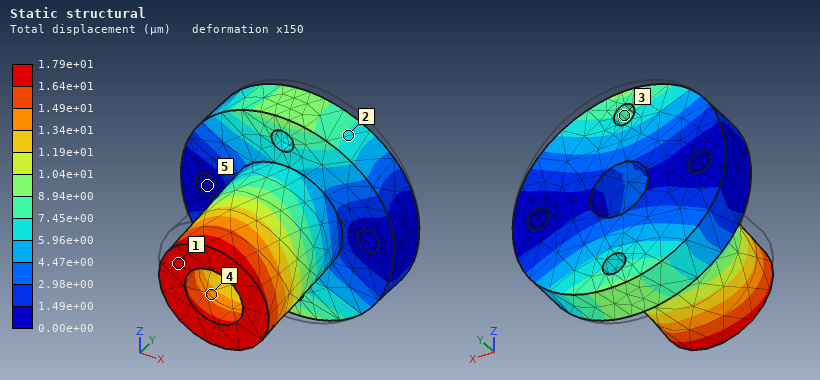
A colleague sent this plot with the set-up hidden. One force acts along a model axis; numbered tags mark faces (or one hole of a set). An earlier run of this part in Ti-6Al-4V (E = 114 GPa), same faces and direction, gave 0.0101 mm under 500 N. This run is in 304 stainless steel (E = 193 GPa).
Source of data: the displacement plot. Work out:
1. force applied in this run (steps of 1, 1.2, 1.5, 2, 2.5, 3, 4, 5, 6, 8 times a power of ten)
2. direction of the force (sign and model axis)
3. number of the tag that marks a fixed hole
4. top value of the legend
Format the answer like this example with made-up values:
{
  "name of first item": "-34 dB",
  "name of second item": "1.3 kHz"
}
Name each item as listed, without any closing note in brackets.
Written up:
{
  "force applied in this run": "1.5 kN",
  "direction of the force": "-Z",
  "number of the tag that marks a fixed hole": "5",
  "top value of the legend": "1.79e+01 µm"
}
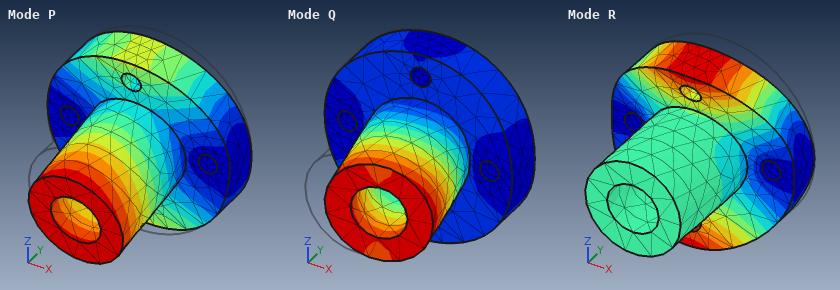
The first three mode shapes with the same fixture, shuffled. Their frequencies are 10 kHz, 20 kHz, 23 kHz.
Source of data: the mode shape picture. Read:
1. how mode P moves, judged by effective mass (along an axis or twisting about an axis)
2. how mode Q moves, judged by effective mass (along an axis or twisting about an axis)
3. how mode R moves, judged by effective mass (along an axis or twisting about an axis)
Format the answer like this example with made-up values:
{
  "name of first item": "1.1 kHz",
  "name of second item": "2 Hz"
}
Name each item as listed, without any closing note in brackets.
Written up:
{
  "how mode P moves, judged by effective mass": "along Z",
  "how mode Q moves, judged by effective mass": "along X",
  "how mode R moves, judged by effective mass": "along Y"
}
